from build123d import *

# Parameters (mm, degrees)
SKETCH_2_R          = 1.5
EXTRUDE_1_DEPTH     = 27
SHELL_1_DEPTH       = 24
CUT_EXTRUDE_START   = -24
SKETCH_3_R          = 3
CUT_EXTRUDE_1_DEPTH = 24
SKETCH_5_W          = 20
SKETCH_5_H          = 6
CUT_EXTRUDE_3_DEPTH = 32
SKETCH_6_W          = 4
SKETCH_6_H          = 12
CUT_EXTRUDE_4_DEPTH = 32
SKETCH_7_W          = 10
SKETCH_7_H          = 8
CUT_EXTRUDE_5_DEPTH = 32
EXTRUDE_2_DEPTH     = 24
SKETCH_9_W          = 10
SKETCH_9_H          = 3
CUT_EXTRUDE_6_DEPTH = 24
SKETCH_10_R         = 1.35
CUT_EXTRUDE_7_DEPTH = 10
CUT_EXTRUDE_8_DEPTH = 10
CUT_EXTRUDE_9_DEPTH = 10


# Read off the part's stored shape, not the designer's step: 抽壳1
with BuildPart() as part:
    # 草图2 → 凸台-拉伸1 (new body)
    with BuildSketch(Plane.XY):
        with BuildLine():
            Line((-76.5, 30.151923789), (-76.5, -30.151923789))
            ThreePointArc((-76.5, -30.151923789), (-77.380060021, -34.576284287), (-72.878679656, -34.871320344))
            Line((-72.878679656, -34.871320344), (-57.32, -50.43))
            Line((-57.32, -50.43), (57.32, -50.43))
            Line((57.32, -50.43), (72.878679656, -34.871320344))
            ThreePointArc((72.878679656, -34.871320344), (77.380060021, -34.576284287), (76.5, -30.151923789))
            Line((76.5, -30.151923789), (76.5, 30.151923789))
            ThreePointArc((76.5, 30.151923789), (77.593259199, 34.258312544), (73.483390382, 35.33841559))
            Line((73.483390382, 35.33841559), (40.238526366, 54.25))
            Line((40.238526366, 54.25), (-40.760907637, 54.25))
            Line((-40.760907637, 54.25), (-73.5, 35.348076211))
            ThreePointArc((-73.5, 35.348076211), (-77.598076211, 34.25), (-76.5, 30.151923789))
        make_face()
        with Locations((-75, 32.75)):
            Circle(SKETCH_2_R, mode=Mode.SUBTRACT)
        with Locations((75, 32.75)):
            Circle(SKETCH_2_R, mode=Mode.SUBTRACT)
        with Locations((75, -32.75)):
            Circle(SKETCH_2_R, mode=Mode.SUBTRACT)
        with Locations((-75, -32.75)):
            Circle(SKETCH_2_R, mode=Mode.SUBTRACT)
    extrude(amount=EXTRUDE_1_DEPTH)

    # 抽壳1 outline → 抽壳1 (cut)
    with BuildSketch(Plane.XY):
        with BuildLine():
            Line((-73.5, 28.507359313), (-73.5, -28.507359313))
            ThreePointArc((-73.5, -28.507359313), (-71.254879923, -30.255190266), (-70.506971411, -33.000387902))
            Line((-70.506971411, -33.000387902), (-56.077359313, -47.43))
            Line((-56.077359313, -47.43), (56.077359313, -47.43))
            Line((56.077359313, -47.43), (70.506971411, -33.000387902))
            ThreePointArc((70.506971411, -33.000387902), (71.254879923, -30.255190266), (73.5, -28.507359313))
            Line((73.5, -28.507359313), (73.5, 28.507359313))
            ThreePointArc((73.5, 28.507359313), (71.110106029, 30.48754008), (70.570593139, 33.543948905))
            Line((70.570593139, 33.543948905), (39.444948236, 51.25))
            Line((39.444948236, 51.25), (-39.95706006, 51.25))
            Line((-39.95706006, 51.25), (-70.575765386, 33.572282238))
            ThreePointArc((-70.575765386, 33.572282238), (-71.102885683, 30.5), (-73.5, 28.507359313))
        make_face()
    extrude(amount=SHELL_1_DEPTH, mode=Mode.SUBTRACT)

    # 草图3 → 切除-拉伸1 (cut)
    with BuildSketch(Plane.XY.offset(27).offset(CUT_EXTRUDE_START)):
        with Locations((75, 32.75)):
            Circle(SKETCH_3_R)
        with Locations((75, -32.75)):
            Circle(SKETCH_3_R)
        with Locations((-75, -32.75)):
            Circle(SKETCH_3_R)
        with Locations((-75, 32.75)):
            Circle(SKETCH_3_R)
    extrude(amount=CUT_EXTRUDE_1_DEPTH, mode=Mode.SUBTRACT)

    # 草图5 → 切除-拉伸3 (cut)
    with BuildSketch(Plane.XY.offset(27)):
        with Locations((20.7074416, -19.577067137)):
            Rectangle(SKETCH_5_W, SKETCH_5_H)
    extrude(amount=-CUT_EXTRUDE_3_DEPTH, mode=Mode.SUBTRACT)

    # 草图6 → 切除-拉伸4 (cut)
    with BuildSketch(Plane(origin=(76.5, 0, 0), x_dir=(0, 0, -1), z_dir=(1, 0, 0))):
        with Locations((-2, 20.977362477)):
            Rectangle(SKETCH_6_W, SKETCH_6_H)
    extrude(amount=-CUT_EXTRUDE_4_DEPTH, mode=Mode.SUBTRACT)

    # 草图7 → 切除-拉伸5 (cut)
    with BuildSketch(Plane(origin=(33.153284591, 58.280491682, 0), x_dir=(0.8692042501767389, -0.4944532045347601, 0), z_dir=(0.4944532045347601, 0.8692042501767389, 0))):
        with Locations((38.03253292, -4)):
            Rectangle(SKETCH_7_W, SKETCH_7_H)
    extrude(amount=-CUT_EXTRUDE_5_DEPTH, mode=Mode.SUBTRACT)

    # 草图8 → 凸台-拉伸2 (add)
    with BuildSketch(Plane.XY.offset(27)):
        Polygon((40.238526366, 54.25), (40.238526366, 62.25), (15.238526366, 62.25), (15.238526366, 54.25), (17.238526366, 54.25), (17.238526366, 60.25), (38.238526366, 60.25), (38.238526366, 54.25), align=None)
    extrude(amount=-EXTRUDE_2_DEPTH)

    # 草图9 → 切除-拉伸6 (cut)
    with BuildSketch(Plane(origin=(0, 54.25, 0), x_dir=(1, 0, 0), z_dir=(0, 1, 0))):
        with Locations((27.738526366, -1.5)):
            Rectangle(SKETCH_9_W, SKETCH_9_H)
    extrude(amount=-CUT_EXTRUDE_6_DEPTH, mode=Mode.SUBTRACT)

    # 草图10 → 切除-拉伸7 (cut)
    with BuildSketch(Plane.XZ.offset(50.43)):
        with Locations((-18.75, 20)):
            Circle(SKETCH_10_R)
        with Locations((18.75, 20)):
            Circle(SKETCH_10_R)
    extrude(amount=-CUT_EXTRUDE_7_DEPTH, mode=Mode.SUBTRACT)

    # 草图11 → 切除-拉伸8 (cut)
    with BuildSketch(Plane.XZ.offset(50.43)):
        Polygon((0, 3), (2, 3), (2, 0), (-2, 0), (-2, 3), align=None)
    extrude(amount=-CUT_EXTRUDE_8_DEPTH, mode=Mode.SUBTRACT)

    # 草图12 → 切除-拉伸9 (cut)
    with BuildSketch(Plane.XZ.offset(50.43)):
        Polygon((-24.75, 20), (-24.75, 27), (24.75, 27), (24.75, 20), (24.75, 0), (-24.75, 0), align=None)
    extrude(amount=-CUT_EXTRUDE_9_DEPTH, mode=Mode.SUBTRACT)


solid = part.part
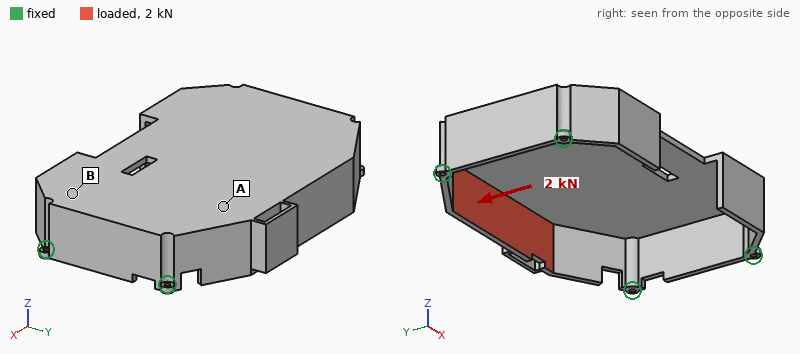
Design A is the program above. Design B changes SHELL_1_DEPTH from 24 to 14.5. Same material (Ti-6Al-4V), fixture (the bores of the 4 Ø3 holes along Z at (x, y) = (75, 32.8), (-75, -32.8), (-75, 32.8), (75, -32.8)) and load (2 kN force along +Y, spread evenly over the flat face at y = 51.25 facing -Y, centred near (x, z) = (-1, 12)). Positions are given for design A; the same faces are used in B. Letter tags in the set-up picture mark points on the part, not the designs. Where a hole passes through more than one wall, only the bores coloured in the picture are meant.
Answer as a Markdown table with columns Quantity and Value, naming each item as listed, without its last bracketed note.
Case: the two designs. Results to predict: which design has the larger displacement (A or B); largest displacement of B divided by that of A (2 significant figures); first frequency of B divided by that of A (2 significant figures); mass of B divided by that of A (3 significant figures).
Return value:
| Quantity | Value |
|---|---|
| which design has the larger displacement | A |
| largest displacement of B divided by that of A | 0.22 |
| first frequency of B divided by that of A | 1.5 |
| mass of B divided by that of A | 2.71 |
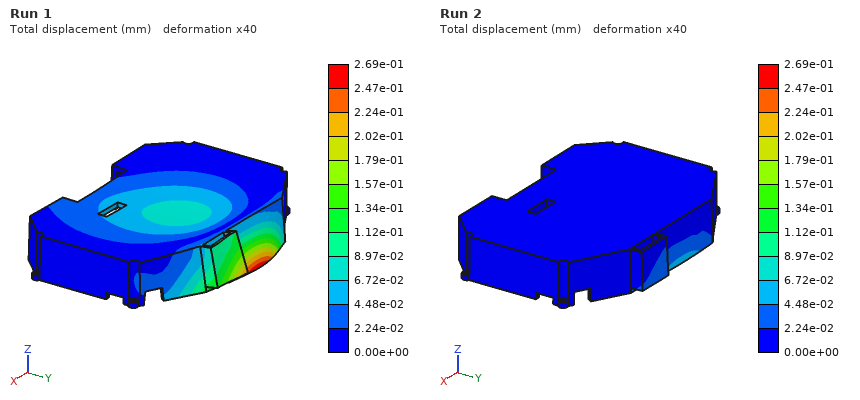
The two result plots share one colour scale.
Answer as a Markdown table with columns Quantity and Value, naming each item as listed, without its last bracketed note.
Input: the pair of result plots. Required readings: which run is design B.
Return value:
| Quantity | Value |
|---|---|
| which run is design B | Run 2 |
